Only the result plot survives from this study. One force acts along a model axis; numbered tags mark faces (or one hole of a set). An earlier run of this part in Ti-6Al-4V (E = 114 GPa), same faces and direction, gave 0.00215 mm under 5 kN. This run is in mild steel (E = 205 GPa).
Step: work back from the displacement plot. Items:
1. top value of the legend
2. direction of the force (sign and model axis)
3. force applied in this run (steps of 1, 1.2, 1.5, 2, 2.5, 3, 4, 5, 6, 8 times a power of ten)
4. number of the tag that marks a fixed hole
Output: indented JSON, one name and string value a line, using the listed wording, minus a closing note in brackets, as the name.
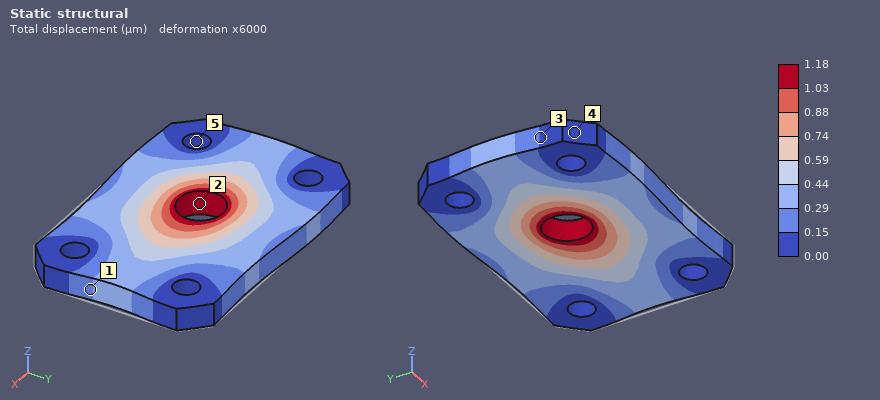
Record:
{
  "top value of the legend": "1.18 µm",
  "direction of the force": "-X",
  "force applied in this run": "5 kN",
  "number of the tag that marks a fixed hole": "5"
}
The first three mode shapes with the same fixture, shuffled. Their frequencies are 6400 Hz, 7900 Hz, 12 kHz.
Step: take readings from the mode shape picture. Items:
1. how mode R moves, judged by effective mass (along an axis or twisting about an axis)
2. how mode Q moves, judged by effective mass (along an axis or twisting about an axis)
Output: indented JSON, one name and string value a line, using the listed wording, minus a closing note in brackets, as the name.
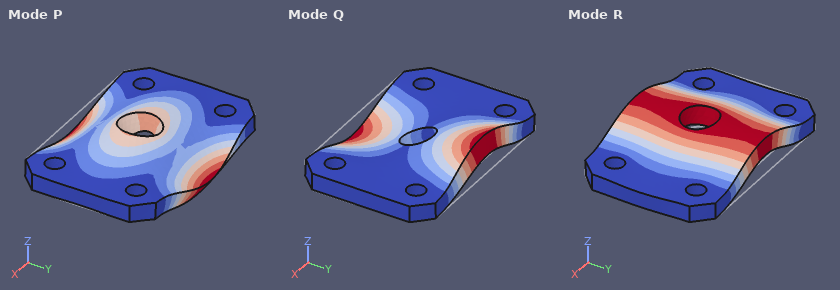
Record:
{
  "how mode R moves, judged by effective mass": "along Z",
  "how mode Q moves, judged by effective mass": "twisting about X"
}
